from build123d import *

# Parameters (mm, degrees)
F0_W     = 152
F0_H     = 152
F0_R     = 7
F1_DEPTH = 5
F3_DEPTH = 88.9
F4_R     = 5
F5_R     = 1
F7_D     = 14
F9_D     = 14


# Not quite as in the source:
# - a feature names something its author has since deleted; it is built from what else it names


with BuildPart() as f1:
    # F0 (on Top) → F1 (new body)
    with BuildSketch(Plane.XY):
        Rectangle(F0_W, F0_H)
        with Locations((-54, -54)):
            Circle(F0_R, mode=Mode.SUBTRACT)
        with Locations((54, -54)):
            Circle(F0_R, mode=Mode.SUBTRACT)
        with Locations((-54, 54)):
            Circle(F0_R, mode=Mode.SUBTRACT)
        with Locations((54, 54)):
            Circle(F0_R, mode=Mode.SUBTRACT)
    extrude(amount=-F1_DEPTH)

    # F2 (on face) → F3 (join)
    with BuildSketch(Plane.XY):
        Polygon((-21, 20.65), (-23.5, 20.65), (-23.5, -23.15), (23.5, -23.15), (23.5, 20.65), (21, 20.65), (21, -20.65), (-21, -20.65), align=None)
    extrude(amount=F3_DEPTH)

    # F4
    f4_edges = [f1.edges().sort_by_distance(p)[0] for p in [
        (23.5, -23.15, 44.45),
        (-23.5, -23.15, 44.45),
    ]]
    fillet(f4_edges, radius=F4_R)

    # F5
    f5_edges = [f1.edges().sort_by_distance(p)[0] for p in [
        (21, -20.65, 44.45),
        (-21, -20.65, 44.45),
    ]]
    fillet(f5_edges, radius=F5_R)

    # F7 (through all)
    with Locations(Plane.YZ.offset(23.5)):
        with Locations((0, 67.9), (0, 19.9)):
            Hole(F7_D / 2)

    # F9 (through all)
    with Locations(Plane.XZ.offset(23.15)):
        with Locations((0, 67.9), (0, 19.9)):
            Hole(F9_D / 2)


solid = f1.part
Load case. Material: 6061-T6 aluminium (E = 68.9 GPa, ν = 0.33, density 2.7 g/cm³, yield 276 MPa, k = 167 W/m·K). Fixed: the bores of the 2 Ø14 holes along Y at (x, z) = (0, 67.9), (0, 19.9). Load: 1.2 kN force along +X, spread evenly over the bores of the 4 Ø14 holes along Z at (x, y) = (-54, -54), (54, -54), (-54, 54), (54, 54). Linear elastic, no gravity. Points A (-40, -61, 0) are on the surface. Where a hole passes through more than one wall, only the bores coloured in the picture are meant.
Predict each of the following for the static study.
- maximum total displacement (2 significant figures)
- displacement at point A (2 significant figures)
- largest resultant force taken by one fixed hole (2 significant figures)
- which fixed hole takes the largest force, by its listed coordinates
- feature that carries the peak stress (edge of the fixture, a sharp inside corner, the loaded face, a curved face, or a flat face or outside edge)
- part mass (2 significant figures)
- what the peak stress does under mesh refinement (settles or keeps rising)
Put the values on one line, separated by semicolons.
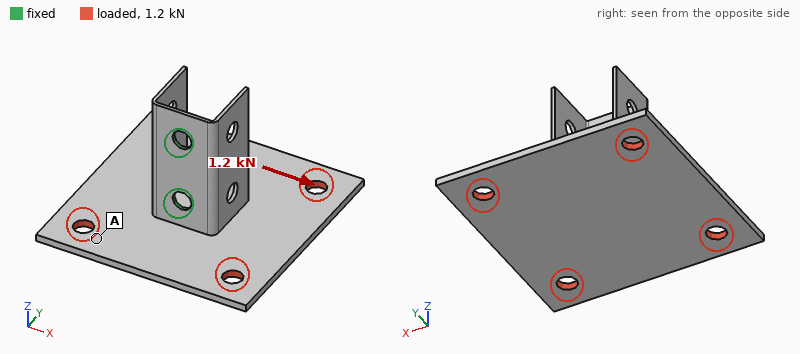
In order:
1.3 mm; 0.57 mm; 1.5 kN; (0, 19.9); edge of the fixture; 370 g; keeps rising
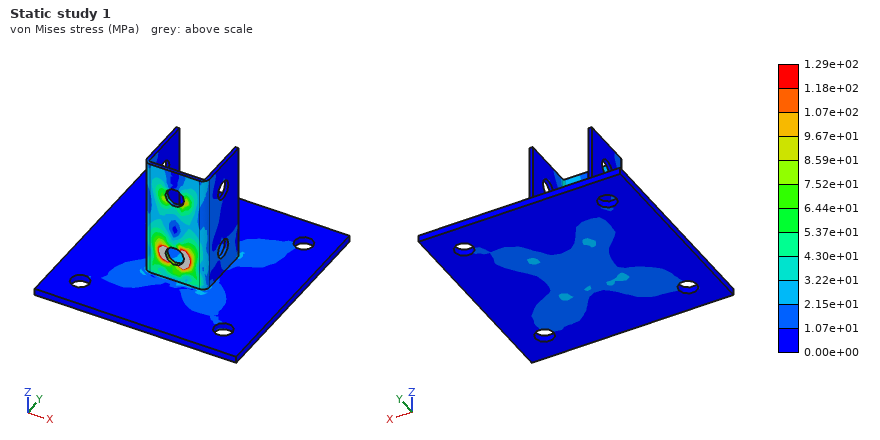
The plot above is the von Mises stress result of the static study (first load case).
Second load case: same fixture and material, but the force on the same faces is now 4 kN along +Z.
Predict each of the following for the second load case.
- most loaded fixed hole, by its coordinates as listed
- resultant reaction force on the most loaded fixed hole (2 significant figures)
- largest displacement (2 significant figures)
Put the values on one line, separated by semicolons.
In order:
(0, 19.9); 2.7 kN; 2.1 mm
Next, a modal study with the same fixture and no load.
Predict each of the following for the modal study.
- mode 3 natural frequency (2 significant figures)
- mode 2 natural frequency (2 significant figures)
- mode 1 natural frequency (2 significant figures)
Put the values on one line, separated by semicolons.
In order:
680 Hz; 480 Hz; 220 Hz
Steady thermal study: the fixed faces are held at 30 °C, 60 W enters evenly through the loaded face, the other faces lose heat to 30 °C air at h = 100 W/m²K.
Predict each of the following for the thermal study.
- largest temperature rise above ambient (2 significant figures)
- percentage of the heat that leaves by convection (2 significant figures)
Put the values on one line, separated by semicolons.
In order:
17 K; 87 %
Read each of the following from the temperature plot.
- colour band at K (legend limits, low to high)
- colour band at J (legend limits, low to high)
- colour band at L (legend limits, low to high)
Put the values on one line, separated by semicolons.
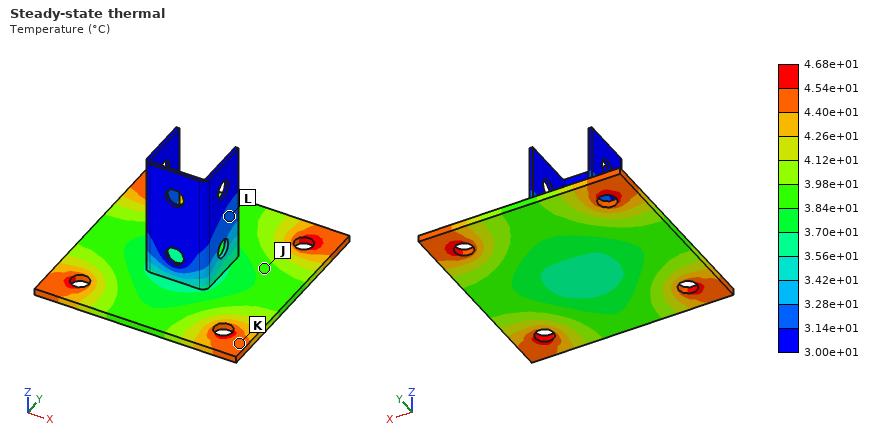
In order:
4.40e+01 to 4.54e+01 °C; 3.84e+01 to 3.98e+01 °C; 3.14e+01 to 3.28e+01 °C
